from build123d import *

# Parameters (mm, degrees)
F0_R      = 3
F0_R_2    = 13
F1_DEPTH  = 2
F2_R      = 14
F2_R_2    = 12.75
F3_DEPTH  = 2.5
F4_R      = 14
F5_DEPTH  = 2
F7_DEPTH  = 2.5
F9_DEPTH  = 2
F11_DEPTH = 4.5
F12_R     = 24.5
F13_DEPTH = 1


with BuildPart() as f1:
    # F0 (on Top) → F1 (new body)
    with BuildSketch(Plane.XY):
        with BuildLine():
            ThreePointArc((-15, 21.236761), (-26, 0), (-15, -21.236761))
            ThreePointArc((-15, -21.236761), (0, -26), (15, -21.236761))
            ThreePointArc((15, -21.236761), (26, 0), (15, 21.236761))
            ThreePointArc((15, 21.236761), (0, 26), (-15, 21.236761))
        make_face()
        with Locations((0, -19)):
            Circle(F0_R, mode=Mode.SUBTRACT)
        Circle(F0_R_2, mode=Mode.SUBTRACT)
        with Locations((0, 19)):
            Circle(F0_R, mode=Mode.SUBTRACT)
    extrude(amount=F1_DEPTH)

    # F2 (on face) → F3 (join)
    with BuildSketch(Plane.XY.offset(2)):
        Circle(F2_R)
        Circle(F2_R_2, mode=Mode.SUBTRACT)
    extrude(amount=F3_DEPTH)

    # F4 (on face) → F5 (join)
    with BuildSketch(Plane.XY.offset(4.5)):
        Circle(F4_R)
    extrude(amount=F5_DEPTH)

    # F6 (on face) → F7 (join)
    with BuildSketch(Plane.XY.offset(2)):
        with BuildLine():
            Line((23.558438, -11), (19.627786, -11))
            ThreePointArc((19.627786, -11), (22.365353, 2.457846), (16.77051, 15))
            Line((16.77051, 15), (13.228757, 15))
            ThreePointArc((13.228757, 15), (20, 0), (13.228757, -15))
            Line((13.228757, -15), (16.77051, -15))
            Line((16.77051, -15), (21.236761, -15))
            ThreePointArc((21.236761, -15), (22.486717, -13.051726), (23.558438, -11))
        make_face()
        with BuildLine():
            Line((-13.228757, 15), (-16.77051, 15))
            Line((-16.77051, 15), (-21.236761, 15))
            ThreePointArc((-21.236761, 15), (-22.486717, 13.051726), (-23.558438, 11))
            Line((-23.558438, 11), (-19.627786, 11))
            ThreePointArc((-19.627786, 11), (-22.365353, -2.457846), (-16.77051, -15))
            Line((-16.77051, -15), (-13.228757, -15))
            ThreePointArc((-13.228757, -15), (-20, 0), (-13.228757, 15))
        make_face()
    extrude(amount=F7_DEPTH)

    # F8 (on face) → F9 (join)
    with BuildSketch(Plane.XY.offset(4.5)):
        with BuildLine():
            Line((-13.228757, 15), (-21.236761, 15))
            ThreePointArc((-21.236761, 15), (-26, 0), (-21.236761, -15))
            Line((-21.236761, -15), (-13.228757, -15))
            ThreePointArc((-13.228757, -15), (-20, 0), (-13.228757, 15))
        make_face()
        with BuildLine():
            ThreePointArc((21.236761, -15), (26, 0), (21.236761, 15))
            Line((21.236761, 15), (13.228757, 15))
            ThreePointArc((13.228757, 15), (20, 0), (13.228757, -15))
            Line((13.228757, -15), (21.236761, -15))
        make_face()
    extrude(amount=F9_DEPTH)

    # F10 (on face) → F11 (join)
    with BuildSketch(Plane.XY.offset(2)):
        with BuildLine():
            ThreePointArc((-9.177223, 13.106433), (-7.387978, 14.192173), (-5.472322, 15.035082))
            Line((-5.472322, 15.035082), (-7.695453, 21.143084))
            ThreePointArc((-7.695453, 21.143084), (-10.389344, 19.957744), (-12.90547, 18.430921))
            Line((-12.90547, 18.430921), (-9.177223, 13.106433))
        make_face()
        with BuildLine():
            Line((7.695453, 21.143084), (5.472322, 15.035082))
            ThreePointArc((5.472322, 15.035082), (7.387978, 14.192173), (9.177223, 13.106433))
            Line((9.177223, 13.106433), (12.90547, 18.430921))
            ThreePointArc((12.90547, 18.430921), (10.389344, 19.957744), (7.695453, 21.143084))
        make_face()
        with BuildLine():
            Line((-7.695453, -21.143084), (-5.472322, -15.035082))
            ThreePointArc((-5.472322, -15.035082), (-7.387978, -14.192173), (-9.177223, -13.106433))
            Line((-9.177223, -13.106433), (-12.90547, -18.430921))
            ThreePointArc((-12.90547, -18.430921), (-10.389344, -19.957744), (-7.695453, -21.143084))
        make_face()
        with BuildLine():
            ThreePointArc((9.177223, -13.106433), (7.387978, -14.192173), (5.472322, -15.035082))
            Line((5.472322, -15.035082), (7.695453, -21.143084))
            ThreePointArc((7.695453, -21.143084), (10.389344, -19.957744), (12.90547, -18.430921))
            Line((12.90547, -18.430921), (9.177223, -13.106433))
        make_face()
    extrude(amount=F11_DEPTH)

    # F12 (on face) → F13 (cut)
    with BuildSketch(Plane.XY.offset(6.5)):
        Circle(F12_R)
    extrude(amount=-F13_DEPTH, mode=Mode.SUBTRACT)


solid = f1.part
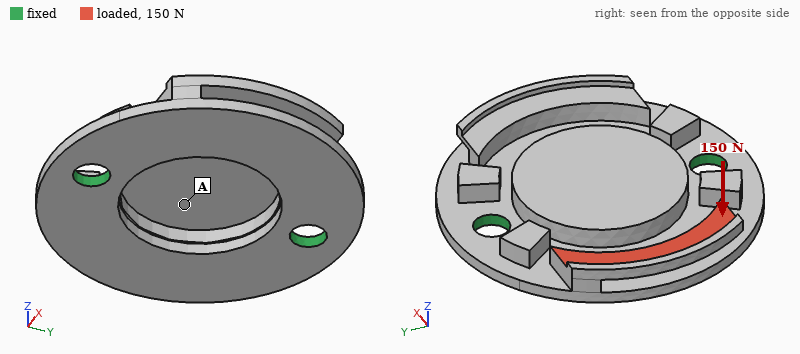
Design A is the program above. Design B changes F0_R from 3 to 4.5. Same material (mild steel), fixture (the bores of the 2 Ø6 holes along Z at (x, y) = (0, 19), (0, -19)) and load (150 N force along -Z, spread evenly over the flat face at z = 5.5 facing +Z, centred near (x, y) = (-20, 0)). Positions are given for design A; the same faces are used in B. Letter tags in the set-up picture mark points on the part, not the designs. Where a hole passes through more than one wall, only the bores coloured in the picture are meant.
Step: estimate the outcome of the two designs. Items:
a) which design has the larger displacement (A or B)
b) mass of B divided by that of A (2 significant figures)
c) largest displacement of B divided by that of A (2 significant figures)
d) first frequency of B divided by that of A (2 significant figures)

A
0.97
0.76
1.3
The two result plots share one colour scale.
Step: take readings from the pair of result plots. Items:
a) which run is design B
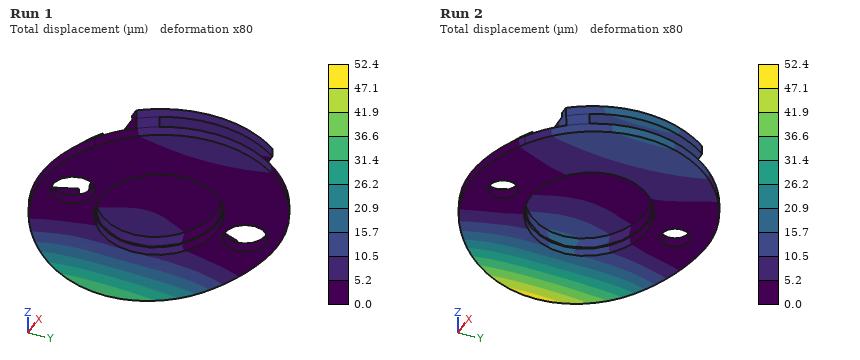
Run 1
